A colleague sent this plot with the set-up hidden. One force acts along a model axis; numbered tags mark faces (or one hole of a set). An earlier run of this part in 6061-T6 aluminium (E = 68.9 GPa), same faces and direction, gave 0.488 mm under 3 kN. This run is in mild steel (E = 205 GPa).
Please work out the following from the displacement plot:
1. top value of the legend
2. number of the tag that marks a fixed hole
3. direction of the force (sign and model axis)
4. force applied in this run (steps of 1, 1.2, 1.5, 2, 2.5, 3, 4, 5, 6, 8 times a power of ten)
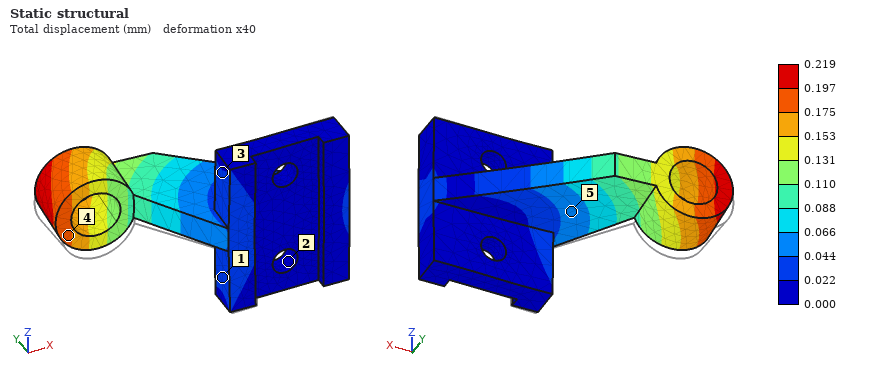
0.219 mm
2
+Y
4 kN
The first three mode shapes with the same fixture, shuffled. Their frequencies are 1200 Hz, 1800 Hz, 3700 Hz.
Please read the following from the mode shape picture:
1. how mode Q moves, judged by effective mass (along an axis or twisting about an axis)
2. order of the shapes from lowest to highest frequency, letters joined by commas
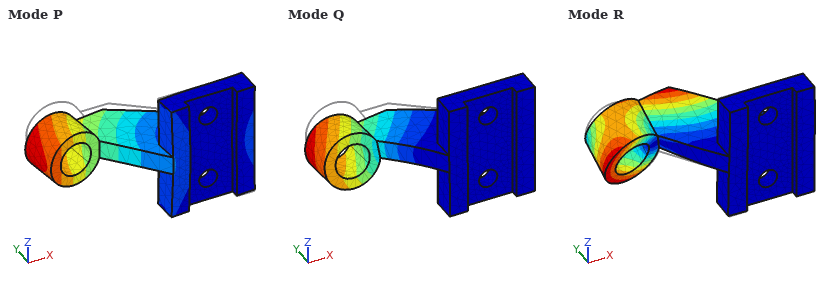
along Z
Q, P, R
